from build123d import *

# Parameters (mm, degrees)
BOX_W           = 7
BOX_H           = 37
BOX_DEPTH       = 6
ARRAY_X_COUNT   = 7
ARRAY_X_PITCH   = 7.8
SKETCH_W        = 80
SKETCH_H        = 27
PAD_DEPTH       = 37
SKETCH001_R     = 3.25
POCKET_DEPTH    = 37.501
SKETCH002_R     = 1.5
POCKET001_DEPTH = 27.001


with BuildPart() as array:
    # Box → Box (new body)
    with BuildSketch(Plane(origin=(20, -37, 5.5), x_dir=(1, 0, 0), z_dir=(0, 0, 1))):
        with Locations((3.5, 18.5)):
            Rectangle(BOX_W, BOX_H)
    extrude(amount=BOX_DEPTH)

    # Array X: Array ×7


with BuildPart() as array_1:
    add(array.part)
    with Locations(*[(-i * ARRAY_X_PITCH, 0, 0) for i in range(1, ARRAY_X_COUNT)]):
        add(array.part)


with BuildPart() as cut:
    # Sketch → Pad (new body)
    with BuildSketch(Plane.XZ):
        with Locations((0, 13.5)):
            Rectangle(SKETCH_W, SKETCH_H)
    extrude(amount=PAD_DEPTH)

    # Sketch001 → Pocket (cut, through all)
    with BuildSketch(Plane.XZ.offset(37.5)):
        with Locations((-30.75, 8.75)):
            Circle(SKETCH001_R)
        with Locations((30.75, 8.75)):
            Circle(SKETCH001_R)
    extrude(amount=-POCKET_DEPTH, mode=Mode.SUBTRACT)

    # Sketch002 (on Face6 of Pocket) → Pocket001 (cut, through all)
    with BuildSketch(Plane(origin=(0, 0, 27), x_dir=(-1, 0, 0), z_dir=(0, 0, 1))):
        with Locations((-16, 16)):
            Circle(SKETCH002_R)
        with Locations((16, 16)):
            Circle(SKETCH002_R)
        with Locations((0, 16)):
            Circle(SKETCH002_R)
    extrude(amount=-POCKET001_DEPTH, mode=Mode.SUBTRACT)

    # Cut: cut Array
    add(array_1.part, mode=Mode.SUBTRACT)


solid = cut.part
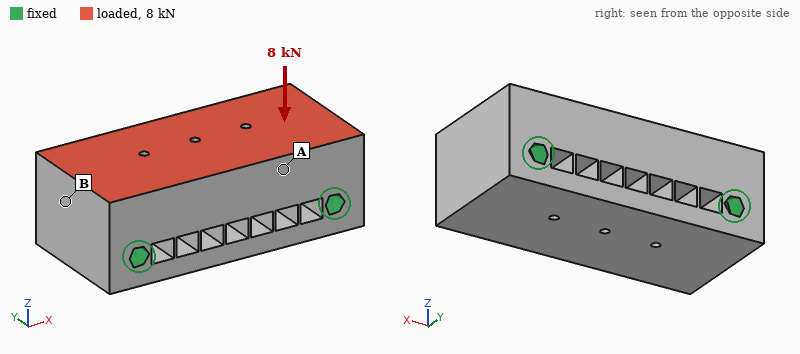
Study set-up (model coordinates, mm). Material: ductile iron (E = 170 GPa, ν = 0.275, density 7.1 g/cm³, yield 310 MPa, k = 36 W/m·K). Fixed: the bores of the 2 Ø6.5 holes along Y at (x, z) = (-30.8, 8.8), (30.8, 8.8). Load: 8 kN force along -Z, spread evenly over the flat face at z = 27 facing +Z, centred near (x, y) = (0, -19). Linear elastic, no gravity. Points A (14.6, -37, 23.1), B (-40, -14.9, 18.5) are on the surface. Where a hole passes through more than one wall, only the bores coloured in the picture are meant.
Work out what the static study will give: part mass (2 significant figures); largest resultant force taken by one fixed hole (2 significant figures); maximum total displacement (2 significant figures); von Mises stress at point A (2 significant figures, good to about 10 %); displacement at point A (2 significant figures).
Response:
470 g
4.3 kN
3.9 µm
7.7 MPa
2.7 µm
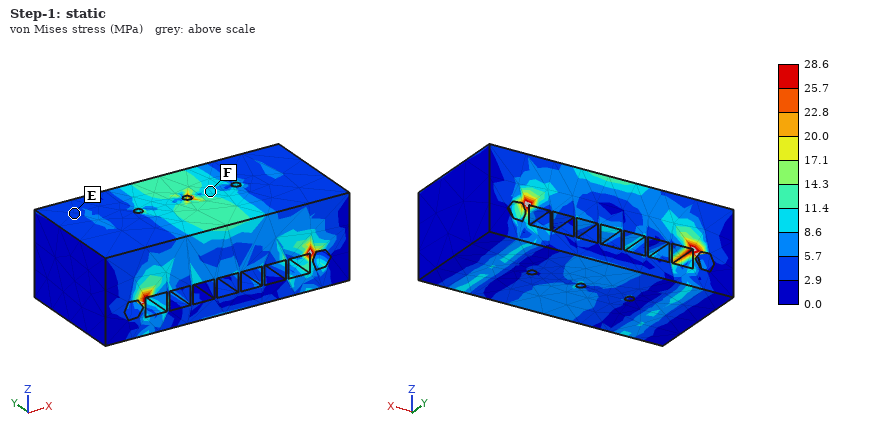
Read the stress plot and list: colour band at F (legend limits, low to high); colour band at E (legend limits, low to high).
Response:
8.6 to 11.4 MPa
2.9 to 5.7 MPa
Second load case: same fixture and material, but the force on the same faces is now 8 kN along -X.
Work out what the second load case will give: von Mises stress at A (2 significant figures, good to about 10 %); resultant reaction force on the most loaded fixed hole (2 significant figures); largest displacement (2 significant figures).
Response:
6.5 MPa
4.3 kN
2.8 µm
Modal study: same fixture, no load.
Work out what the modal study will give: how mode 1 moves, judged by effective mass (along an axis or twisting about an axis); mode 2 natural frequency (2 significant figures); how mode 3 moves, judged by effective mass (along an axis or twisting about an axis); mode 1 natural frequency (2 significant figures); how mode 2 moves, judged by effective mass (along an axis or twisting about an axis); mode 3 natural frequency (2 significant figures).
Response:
along Z
17 kHz
along Y
12 kHz
along Y
18 kHz
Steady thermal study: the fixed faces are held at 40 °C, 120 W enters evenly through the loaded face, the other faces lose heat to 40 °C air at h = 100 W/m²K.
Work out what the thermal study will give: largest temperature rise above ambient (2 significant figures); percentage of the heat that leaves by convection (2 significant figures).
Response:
42 K
19 %
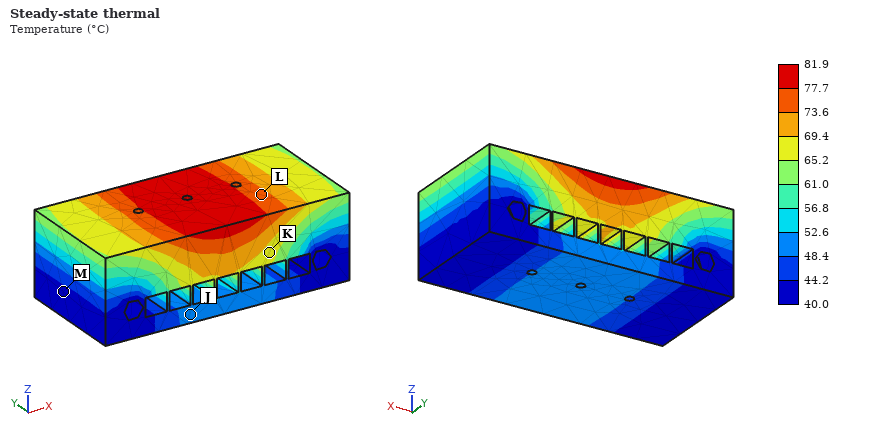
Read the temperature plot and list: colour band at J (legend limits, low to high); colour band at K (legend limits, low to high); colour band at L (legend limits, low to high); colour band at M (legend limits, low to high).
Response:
48.4 to 52.6 °C
65.2 to 69.4 °C
73.6 to 77.7 °C
40.0 to 44.2 °C
